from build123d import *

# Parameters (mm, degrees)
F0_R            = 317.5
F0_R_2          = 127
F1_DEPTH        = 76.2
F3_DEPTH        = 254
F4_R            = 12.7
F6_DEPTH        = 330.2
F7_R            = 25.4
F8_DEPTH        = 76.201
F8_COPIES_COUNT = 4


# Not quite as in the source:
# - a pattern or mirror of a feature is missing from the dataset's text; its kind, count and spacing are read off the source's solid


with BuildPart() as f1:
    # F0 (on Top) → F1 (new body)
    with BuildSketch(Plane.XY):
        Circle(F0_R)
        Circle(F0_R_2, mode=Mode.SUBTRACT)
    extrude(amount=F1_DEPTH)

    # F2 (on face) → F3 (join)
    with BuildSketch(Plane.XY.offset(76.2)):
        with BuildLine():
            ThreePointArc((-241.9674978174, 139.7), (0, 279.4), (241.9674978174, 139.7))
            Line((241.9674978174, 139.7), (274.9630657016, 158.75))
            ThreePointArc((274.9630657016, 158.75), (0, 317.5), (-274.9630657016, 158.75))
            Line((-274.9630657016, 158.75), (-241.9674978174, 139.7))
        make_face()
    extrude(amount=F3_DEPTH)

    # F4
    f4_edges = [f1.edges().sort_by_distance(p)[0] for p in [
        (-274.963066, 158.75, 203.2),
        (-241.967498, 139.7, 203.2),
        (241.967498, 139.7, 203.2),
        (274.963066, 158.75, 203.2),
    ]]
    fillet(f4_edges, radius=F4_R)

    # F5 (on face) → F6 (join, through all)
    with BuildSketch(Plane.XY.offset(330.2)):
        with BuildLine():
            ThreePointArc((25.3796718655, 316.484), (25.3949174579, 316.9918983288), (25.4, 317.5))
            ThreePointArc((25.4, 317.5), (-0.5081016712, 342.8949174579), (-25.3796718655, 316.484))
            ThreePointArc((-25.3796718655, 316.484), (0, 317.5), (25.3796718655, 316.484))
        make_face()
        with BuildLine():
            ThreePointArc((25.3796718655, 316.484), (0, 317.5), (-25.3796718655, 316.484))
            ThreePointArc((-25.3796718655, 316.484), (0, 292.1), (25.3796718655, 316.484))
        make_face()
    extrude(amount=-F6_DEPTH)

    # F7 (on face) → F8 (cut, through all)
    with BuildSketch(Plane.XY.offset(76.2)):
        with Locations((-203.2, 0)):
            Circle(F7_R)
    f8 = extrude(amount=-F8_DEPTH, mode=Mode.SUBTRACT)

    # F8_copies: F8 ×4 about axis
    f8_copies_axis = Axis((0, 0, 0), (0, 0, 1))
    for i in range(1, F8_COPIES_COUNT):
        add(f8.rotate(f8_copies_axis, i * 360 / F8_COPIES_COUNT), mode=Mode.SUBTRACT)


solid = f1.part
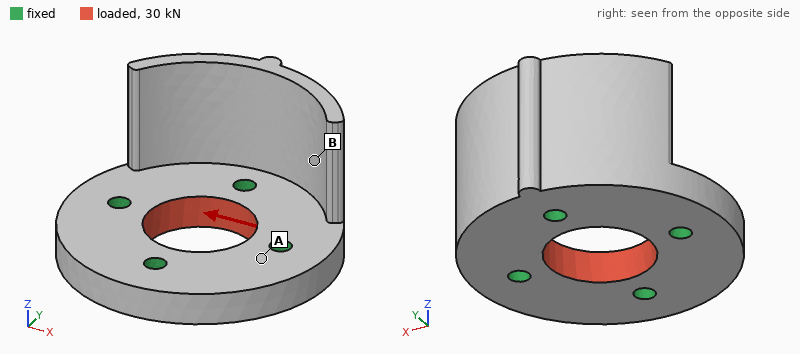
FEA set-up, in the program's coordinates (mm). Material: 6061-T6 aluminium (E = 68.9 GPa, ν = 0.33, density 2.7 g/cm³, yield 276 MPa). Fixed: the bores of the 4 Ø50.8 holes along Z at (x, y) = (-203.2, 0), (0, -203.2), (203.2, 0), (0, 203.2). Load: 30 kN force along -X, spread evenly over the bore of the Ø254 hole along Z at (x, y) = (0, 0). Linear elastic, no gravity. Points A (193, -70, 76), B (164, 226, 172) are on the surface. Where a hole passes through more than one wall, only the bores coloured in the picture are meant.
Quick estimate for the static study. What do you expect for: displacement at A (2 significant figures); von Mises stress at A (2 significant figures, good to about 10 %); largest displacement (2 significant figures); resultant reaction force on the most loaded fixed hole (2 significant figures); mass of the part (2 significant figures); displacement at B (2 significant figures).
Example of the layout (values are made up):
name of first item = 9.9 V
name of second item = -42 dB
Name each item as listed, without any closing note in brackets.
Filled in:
displacement at A = 0.62 µm
von Mises stress at A = 0.39 MPa
largest displacement = 1.4 µm
resultant reaction force on the most loaded fixed hole = 7.7 kN
mass of the part = 70 kg
displacement at B = 0.56 µm
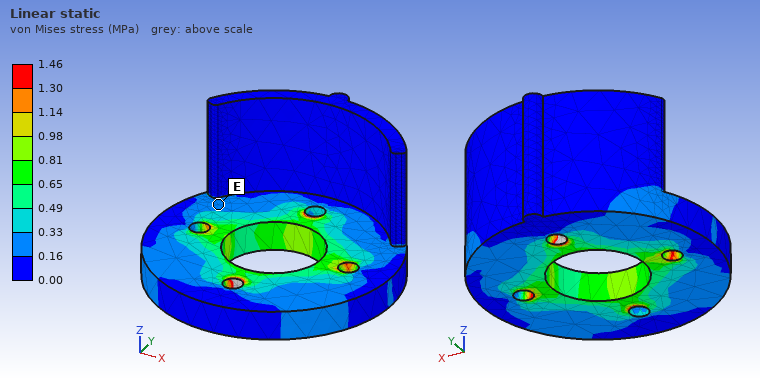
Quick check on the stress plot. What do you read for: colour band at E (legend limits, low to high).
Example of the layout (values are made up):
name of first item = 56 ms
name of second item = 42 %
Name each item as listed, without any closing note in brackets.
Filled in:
colour band at E = 0.16 to 0.33 MPa
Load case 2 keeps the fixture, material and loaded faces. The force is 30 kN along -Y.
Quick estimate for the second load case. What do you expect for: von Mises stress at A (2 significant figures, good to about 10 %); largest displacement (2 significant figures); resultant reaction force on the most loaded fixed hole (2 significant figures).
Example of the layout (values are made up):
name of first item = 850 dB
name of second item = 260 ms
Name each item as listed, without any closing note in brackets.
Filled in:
von Mises stress at A = 0.40 MPa
largest displacement = 1.4 µm
resultant reaction force on the most loaded fixed hole = 7.7 kN
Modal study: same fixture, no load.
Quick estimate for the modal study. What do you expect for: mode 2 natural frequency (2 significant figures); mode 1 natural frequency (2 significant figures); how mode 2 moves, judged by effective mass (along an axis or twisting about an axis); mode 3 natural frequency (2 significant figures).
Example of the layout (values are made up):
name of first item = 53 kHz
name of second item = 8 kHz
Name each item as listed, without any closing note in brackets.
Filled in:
mode 2 natural frequency = 690 Hz
mode 1 natural frequency = 530 Hz
how mode 2 moves, judged by effective mass = along Y
mode 3 natural frequency = 910 Hz
